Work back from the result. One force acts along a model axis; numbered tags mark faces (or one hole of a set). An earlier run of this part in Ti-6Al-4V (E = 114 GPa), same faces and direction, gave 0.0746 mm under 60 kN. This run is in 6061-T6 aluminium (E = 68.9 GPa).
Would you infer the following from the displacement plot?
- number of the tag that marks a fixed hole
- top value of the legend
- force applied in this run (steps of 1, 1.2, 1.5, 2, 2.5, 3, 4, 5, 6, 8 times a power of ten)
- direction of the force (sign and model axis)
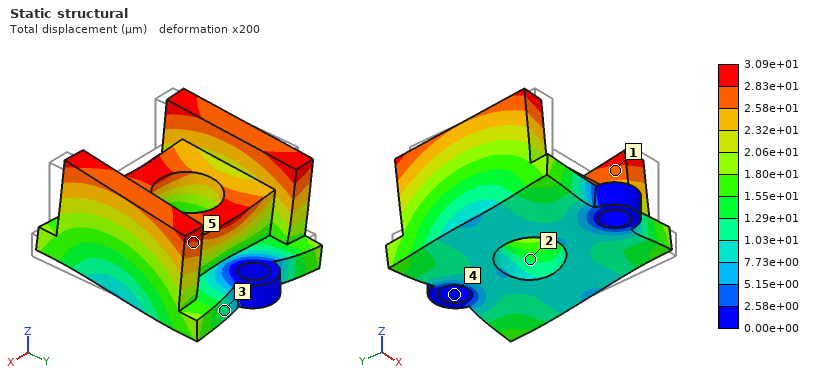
4
3.09e+01 µm
15 kN
+Y
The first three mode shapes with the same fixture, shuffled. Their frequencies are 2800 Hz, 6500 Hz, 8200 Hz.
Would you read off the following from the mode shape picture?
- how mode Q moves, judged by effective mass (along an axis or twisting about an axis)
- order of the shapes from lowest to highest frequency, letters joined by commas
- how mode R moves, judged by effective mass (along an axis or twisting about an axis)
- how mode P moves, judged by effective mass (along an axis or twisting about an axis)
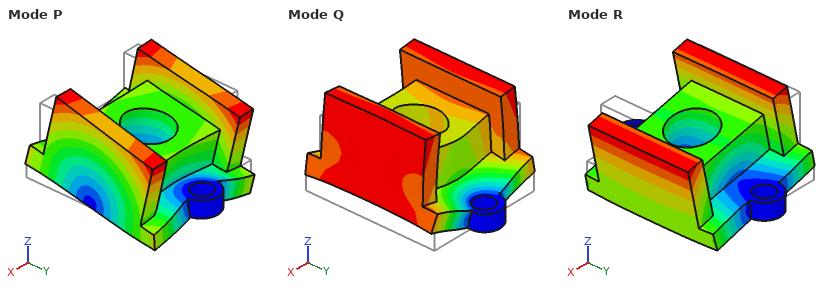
along Z
R, Q, P
along X
along Y
